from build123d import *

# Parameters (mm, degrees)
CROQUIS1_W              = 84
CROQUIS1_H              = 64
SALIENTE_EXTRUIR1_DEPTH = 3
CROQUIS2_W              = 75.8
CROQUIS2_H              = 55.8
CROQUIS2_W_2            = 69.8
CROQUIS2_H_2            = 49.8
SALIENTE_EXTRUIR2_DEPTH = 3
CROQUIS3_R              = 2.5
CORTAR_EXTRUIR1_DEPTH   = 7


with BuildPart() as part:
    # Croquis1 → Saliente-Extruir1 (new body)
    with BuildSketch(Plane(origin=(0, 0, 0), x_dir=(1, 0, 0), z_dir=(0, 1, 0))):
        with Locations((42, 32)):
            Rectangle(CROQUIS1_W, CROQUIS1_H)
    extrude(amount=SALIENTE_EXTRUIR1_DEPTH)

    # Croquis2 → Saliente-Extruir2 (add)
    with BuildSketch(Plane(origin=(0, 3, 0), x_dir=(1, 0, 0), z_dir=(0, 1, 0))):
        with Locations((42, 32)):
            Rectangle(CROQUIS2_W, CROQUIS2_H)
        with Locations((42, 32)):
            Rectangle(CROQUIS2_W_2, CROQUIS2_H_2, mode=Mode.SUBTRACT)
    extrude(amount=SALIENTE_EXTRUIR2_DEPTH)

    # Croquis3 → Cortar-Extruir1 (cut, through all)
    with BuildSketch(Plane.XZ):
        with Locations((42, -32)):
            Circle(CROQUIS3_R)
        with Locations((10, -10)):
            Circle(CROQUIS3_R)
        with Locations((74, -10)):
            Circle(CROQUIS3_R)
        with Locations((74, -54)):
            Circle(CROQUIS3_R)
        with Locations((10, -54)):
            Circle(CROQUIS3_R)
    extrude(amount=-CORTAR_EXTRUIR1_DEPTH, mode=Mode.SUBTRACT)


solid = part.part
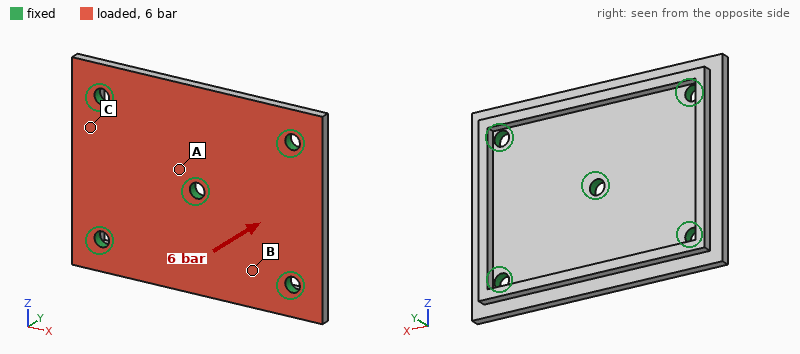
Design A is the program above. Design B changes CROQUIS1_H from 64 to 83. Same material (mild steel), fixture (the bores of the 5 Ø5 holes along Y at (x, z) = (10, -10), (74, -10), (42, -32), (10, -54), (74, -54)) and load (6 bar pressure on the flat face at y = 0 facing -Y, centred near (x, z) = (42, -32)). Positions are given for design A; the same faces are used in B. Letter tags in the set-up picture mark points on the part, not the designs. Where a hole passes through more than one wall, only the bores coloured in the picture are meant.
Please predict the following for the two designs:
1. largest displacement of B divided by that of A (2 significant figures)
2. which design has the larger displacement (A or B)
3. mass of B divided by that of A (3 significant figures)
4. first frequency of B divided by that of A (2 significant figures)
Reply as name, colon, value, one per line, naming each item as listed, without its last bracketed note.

largest displacement of B divided by that of A: 2.8
which design has the larger displacement: B
mass of B divided by that of A: 1.26
first frequency of B divided by that of A: 0.68
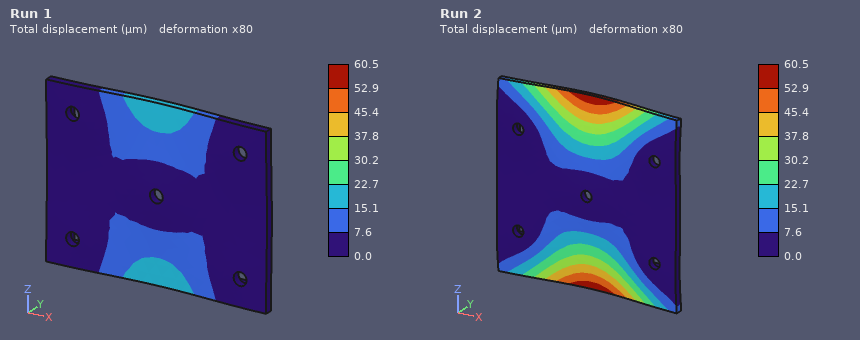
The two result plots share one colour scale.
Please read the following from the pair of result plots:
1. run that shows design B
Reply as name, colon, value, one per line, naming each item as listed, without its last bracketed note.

run that shows design B: Run 2
